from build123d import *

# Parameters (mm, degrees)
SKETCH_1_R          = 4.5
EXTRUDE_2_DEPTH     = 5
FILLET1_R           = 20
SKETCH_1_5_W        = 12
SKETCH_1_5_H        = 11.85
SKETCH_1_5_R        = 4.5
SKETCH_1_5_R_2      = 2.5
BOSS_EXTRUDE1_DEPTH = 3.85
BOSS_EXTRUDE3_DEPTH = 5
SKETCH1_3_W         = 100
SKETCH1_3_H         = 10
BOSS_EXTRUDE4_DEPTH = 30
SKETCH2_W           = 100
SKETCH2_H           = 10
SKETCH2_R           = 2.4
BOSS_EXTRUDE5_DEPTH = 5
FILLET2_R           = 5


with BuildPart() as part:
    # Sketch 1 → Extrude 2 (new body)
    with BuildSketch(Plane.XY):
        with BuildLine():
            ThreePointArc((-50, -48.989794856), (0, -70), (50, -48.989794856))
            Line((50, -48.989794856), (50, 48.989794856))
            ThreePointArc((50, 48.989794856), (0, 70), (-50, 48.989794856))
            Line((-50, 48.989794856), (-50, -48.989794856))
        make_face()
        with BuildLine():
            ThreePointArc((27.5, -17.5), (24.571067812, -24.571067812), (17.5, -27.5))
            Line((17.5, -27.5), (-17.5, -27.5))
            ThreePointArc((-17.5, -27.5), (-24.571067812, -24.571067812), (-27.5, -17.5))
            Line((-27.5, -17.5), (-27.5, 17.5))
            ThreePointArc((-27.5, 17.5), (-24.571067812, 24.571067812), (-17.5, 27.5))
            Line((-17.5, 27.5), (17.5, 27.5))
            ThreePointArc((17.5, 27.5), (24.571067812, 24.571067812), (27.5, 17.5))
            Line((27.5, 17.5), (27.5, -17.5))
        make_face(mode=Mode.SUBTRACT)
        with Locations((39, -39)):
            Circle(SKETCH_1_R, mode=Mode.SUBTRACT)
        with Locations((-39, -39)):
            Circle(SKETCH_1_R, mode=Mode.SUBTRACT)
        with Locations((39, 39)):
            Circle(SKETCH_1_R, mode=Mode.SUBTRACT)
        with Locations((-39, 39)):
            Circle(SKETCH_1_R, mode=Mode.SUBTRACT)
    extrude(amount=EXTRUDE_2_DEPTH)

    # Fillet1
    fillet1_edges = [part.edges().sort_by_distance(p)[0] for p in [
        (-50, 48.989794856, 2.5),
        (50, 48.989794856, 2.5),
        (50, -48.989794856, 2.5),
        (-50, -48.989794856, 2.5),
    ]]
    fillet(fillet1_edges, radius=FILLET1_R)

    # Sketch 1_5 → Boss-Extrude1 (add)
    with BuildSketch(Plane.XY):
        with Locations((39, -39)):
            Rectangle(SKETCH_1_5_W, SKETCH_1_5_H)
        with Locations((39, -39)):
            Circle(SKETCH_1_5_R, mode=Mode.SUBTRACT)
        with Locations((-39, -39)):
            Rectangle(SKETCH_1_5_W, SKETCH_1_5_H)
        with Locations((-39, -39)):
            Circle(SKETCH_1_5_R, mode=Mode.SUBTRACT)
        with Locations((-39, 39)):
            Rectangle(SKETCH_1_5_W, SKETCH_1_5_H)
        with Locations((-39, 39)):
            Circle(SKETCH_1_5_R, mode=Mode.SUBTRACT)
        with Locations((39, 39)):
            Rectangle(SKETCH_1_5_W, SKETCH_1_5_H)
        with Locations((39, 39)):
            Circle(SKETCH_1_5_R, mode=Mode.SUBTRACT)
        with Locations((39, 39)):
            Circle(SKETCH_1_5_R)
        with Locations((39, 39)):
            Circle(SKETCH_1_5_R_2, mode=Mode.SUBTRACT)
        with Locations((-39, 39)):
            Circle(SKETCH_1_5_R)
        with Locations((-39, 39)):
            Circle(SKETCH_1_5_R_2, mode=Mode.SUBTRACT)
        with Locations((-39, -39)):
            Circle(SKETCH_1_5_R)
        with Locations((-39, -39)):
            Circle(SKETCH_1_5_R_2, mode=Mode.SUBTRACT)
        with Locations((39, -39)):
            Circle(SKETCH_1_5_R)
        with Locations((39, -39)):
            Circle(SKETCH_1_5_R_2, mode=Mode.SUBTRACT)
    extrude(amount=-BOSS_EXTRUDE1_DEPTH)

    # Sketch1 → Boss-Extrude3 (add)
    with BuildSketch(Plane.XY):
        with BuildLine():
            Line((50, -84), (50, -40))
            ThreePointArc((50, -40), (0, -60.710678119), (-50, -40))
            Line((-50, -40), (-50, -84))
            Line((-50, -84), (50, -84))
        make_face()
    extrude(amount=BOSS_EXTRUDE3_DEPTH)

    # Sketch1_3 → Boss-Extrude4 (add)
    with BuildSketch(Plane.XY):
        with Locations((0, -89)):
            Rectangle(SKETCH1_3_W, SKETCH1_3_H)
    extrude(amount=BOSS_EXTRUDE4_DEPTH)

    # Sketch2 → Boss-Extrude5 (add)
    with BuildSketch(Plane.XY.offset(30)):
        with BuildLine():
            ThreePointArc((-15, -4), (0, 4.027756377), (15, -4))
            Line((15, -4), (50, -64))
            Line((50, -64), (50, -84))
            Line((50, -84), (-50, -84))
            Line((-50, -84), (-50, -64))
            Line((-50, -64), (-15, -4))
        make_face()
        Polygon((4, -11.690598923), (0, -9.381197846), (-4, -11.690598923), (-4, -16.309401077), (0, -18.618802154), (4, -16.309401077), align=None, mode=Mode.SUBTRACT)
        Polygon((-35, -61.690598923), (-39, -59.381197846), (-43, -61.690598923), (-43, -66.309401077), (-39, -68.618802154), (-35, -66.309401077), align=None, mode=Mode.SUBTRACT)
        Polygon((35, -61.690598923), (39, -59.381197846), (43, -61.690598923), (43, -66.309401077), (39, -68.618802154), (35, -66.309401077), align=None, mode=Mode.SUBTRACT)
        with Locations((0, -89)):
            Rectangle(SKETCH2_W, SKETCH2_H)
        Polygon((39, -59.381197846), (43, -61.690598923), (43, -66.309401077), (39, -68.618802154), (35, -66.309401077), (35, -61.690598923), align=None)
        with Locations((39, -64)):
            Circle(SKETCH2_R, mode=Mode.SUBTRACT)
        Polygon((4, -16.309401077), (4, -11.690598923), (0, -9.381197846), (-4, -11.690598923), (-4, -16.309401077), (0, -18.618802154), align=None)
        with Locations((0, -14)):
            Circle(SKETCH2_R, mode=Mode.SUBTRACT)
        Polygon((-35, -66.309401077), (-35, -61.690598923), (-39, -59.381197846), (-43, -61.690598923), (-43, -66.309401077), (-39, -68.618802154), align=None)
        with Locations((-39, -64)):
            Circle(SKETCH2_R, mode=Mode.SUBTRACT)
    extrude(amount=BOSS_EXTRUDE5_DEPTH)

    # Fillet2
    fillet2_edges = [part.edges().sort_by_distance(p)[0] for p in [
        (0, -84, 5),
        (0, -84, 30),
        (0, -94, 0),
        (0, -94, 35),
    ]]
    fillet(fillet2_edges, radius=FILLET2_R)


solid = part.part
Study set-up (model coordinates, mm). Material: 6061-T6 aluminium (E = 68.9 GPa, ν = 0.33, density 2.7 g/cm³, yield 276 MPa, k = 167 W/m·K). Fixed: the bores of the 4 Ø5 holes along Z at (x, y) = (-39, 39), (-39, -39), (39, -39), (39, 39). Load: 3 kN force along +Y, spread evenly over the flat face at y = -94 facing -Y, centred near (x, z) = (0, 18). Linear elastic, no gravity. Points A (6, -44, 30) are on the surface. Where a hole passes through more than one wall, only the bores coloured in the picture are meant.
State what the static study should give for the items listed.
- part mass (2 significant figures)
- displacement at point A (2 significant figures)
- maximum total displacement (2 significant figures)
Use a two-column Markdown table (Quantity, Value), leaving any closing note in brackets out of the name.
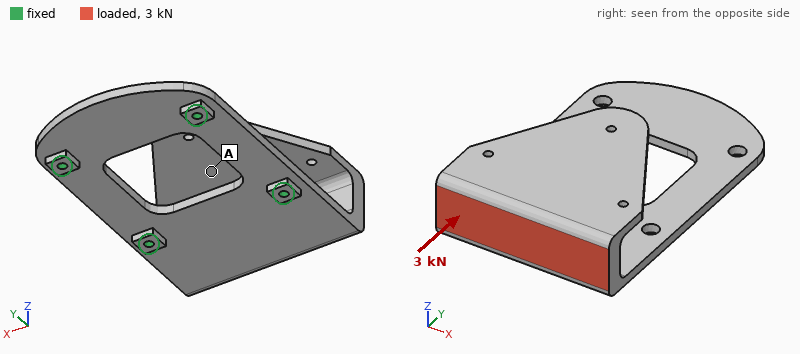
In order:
| Quantity | Value |
|---|---|
| part mass | 340 g |
| displacement at point A | 1.0 mm |
| maximum total displacement | 2.3 mm |
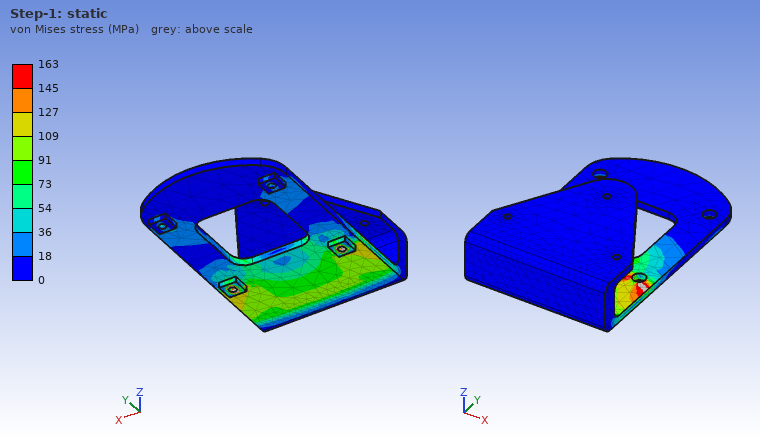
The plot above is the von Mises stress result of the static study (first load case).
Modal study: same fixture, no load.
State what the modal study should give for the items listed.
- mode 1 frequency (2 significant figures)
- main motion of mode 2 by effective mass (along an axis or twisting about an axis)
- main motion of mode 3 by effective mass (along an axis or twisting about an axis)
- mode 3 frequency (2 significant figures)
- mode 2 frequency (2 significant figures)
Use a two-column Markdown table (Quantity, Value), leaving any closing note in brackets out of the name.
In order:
| Quantity | Value |
|---|---|
| mode 1 frequency | 370 Hz |
| main motion of mode 2 by effective mass | along Z |
| main motion of mode 3 by effective mass | along X |
| mode 3 frequency | 850 Hz |
| mode 2 frequency | 690 Hz |
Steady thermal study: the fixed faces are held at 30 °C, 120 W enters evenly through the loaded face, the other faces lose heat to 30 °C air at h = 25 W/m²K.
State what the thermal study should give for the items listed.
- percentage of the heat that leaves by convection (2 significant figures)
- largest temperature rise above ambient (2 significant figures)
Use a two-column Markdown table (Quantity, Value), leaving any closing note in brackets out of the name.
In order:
| Quantity | Value |
|---|---|
| percentage of the heat that leaves by convection | 36 % |
| largest temperature rise above ambient | 72 K |
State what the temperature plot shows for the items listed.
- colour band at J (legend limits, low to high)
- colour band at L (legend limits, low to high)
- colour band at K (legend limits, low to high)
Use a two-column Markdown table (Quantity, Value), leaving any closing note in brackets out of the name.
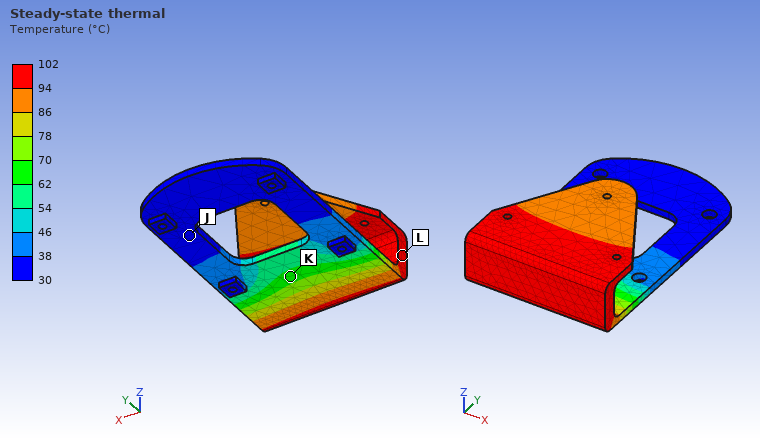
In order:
| Quantity | Value |
|---|---|
| colour band at J | 30 to 38 °C |
| colour band at L | 94 to 102 °C |
| colour band at K | 62 to 70 °C |
